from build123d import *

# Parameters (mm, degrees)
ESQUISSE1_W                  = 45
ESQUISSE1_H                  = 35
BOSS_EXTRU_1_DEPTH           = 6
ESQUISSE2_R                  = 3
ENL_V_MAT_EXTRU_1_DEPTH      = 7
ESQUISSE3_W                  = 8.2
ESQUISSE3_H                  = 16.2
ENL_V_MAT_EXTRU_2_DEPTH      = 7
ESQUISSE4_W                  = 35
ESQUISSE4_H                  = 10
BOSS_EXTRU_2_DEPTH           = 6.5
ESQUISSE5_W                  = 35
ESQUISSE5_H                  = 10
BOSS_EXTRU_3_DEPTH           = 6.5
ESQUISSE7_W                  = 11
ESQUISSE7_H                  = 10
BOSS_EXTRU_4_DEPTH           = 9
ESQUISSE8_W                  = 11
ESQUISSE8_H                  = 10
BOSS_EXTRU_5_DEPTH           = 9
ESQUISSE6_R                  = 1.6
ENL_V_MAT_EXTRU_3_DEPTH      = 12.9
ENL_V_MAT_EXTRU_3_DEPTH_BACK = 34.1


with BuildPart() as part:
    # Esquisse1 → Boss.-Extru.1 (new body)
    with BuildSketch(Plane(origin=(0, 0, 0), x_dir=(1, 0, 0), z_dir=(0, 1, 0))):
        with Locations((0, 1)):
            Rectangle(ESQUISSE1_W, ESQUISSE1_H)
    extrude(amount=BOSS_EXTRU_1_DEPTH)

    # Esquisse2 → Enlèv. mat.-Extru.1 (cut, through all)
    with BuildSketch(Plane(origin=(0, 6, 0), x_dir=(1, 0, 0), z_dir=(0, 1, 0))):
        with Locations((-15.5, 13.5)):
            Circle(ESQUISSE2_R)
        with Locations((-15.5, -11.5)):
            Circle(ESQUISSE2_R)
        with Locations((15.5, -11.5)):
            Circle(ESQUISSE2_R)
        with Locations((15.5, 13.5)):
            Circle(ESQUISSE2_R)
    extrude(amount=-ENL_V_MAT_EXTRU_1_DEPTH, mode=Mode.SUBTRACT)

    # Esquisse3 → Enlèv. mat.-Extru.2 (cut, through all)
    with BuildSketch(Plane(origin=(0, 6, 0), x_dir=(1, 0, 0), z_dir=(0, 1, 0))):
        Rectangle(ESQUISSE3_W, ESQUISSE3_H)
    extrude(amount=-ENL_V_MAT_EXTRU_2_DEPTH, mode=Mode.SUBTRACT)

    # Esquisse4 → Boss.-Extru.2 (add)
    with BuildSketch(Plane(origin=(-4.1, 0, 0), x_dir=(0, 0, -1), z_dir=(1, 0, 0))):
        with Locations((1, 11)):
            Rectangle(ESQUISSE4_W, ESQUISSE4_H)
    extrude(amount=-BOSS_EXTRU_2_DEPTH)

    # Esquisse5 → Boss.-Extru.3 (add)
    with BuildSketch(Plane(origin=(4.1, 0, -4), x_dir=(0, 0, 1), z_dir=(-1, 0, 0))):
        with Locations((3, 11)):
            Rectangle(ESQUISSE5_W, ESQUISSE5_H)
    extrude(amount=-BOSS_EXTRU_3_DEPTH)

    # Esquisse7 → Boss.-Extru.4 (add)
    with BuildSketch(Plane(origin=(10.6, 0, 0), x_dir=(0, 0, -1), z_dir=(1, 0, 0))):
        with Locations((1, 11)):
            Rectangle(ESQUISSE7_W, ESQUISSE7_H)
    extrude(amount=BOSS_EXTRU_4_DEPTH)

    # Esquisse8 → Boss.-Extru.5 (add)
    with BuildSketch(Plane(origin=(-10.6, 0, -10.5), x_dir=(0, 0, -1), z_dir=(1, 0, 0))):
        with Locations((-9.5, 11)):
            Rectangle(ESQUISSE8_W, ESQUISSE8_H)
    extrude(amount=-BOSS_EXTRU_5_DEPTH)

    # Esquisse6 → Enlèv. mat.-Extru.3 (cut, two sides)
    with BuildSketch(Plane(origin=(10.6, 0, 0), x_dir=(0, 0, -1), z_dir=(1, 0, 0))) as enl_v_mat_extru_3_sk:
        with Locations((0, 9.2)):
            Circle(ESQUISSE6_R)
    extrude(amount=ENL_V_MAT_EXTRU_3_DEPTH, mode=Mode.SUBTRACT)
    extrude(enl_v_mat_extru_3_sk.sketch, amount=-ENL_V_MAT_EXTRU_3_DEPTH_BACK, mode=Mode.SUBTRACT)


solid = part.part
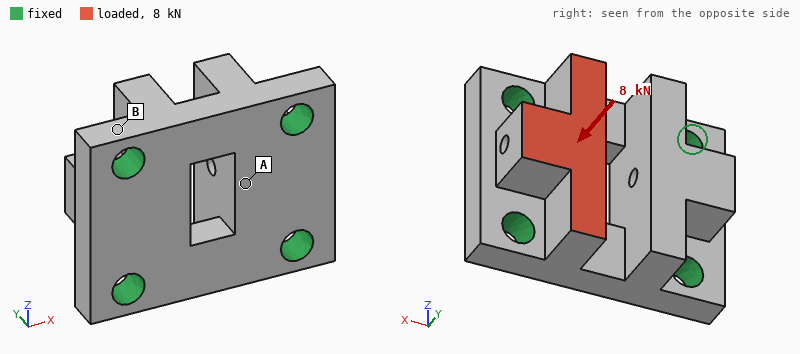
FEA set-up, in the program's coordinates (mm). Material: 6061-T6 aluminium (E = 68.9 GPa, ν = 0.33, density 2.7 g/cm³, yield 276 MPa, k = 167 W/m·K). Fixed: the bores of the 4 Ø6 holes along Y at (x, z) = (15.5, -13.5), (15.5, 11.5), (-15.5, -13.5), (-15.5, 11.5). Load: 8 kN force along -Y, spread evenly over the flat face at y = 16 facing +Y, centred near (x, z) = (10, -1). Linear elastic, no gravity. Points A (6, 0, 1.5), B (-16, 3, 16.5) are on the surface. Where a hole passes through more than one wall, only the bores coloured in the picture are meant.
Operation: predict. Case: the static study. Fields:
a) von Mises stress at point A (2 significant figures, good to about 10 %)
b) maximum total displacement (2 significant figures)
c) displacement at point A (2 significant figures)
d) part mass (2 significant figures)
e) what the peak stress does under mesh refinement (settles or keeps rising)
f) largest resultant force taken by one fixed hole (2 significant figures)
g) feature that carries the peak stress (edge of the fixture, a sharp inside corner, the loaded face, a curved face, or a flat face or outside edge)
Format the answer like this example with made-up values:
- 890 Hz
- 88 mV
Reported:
- 30 MPa
- 30 µm
- 20 µm
- 38 g
- keeps rising
- 3.6 kN
- edge of the fixture
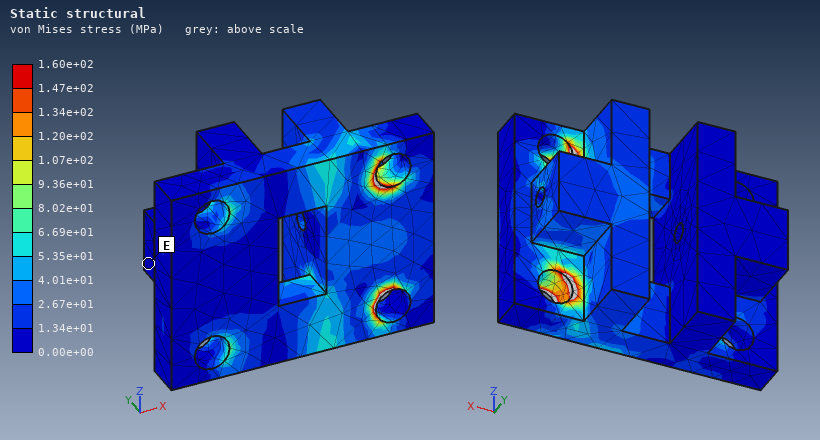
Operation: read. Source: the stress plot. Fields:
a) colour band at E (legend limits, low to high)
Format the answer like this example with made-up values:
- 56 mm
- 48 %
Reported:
- 0.00e+00 to 1.34e+01 MPa
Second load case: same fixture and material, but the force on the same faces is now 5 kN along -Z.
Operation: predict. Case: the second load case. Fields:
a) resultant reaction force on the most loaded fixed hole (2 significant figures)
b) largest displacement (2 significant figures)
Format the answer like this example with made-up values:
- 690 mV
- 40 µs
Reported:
- 3.3 kN
- 28 µm
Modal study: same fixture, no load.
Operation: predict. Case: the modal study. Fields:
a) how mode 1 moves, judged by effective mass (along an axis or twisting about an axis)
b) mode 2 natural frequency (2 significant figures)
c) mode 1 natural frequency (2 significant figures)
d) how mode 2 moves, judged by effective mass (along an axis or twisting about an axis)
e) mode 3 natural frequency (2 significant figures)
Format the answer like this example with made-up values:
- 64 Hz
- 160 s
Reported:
- along Y
- 25 kHz
- 17 kHz
- along X
- 27 kHz
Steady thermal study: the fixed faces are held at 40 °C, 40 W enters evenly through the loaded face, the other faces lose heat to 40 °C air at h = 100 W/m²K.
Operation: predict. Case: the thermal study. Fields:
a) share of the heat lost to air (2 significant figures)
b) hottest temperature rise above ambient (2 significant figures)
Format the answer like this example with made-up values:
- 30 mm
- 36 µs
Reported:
- 4.5 %
- 14 K
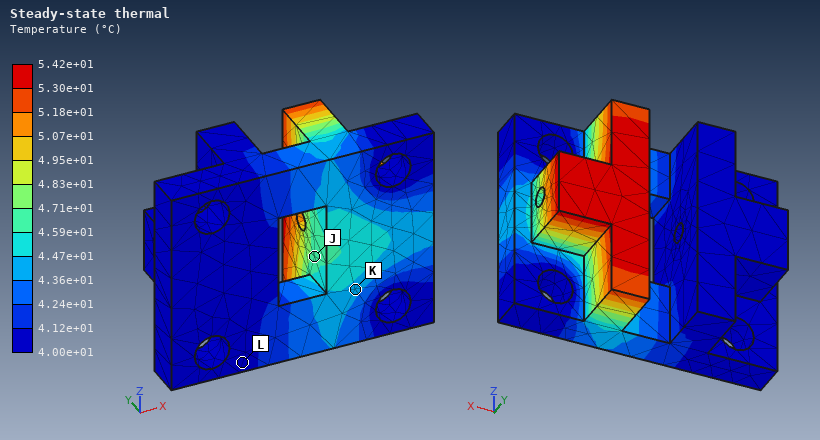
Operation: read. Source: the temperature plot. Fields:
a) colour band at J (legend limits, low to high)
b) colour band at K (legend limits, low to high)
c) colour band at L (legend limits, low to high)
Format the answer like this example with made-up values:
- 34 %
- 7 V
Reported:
- 4.59e+01 to 4.71e+01 °C
- 4.36e+01 to 4.47e+01 °C
- 4.00e+01 to 4.12e+01 °C
